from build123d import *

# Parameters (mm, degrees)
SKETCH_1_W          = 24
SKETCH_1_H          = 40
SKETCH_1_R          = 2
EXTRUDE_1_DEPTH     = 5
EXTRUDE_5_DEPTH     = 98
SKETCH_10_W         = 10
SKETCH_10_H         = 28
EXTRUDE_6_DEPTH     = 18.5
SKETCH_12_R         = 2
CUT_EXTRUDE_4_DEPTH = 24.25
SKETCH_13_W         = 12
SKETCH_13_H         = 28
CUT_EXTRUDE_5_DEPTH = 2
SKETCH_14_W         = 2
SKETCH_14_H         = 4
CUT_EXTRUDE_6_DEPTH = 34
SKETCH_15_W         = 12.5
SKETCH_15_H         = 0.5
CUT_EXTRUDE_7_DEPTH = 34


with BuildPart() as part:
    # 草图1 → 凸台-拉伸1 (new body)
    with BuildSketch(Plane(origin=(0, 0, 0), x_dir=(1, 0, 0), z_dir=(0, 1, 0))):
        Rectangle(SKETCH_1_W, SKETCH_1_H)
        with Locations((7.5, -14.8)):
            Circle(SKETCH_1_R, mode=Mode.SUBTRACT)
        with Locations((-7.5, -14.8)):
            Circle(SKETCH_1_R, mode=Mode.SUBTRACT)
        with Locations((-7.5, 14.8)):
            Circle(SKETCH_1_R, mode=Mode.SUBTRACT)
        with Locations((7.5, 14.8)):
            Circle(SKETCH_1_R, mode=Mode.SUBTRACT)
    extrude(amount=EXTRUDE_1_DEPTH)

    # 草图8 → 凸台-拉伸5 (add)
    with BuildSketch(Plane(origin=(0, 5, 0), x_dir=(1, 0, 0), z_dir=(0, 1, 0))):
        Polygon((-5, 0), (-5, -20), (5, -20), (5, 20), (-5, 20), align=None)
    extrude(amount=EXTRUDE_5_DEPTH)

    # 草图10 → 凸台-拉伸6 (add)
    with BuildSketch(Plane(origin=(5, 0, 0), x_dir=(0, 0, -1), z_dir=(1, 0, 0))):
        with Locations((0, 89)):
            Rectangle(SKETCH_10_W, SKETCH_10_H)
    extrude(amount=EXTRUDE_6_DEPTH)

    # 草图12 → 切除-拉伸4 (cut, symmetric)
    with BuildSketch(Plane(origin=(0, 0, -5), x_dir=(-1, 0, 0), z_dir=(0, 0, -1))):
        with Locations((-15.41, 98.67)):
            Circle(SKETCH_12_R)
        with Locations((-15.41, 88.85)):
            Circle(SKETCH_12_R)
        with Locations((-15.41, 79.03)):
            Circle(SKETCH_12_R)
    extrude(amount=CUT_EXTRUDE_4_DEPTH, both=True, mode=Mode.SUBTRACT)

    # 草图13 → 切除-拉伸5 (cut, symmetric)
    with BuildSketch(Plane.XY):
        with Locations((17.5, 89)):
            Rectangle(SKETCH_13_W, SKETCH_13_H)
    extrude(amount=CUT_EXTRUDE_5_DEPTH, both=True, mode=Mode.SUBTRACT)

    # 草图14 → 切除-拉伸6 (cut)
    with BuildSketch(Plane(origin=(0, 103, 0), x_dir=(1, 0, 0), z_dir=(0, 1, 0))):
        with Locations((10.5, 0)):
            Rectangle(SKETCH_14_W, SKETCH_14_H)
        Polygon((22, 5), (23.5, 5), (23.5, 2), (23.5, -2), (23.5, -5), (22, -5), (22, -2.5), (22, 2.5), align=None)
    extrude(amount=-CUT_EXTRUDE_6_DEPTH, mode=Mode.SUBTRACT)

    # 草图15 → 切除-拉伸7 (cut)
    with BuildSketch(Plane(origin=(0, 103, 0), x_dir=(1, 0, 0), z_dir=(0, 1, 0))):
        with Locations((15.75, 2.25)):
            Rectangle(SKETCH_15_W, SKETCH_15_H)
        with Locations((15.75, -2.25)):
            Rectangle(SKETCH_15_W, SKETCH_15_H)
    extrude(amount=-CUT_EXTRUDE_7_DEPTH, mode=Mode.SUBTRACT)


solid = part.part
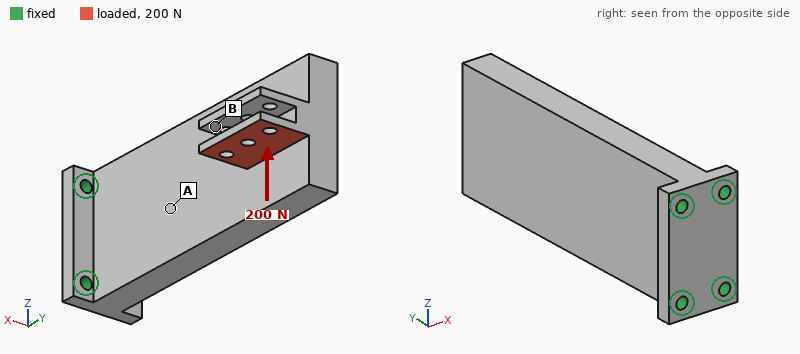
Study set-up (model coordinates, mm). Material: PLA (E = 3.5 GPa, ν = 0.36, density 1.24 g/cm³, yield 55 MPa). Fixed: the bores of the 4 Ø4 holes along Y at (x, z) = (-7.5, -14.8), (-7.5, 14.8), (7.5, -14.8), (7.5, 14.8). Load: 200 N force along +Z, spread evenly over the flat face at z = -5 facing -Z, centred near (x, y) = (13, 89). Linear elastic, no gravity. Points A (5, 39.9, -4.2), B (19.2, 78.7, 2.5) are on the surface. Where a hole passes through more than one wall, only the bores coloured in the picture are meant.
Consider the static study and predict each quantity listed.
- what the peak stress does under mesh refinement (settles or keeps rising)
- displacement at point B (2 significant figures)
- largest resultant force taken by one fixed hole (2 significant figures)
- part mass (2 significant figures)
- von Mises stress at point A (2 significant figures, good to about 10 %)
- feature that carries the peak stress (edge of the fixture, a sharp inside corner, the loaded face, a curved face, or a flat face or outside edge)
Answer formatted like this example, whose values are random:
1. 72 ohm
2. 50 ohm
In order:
1. keeps rising
2. 0.54 mm
3. 360 N
4. 58 g
5. 5.2 MPa
6. edge of the fixture
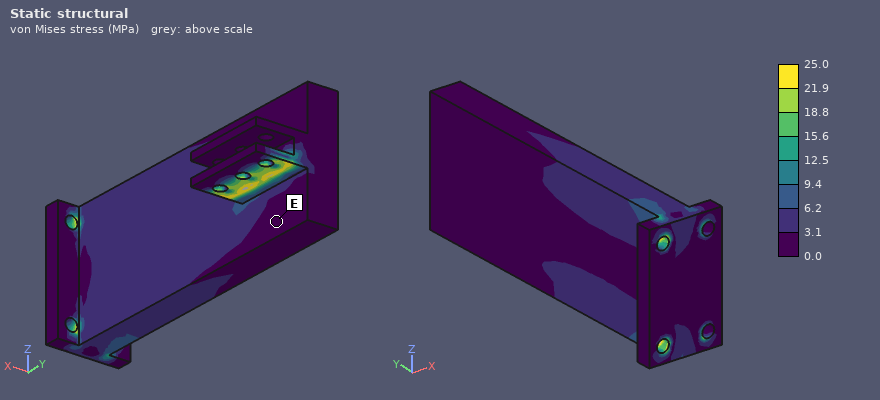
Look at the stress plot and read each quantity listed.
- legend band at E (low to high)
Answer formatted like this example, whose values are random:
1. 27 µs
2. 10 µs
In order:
1. 0.0 to 3.1 MPa
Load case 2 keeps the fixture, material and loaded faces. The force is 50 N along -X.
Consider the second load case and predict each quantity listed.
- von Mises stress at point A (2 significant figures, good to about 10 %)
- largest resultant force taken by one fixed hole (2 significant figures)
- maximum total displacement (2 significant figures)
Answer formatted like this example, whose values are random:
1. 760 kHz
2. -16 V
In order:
1. 3.7 MPa
2. 170 N
3. 1.3 mm
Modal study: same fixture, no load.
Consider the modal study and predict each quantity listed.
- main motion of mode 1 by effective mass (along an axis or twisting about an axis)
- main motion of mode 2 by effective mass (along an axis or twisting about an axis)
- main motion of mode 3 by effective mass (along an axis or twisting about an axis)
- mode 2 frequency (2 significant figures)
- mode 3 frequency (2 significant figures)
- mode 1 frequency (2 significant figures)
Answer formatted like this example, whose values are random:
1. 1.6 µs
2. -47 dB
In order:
1. along X
2. along Z
3. twisting about Y
4. 770 Hz
5. 1200 Hz
6. 230 Hz
